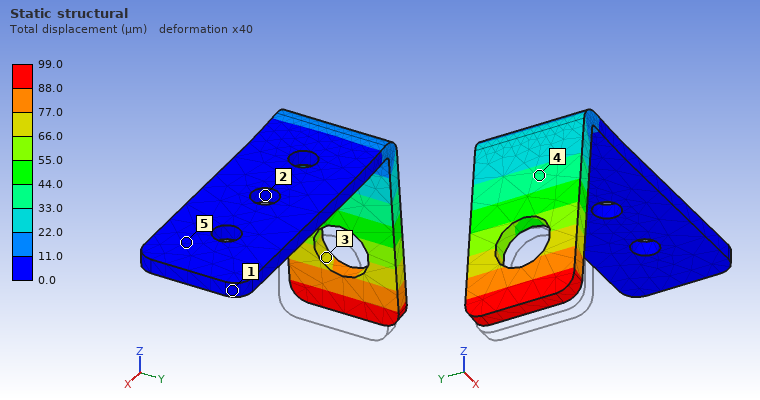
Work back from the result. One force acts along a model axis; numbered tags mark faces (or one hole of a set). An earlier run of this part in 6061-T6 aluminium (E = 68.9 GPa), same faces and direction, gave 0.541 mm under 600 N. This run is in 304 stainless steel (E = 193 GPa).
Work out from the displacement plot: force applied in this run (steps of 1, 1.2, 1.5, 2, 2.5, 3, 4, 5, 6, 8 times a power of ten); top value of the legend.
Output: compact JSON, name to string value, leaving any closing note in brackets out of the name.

{"force applied in this run": "300 N", "top value of the legend": "99.0 µm"}
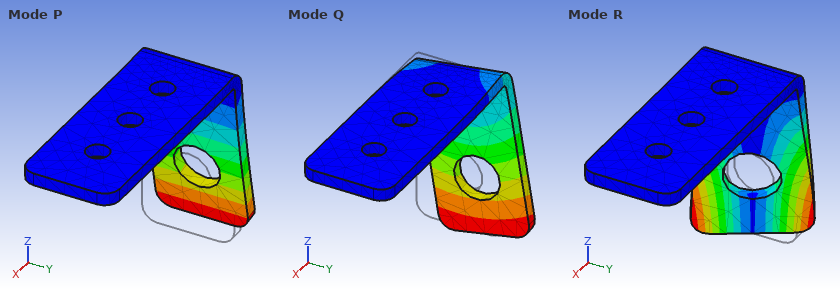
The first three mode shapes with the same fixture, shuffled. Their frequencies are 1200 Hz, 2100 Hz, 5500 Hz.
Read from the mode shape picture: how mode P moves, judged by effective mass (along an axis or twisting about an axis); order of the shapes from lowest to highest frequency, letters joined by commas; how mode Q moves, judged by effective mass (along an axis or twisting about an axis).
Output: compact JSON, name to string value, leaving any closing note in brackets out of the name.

{"how mode P moves, judged by effective mass": "along X", "order of the shapes from lowest to highest frequency, letters joined by commas": "P, Q, R", "how mode Q moves, judged by effective mass": "along Y"}
